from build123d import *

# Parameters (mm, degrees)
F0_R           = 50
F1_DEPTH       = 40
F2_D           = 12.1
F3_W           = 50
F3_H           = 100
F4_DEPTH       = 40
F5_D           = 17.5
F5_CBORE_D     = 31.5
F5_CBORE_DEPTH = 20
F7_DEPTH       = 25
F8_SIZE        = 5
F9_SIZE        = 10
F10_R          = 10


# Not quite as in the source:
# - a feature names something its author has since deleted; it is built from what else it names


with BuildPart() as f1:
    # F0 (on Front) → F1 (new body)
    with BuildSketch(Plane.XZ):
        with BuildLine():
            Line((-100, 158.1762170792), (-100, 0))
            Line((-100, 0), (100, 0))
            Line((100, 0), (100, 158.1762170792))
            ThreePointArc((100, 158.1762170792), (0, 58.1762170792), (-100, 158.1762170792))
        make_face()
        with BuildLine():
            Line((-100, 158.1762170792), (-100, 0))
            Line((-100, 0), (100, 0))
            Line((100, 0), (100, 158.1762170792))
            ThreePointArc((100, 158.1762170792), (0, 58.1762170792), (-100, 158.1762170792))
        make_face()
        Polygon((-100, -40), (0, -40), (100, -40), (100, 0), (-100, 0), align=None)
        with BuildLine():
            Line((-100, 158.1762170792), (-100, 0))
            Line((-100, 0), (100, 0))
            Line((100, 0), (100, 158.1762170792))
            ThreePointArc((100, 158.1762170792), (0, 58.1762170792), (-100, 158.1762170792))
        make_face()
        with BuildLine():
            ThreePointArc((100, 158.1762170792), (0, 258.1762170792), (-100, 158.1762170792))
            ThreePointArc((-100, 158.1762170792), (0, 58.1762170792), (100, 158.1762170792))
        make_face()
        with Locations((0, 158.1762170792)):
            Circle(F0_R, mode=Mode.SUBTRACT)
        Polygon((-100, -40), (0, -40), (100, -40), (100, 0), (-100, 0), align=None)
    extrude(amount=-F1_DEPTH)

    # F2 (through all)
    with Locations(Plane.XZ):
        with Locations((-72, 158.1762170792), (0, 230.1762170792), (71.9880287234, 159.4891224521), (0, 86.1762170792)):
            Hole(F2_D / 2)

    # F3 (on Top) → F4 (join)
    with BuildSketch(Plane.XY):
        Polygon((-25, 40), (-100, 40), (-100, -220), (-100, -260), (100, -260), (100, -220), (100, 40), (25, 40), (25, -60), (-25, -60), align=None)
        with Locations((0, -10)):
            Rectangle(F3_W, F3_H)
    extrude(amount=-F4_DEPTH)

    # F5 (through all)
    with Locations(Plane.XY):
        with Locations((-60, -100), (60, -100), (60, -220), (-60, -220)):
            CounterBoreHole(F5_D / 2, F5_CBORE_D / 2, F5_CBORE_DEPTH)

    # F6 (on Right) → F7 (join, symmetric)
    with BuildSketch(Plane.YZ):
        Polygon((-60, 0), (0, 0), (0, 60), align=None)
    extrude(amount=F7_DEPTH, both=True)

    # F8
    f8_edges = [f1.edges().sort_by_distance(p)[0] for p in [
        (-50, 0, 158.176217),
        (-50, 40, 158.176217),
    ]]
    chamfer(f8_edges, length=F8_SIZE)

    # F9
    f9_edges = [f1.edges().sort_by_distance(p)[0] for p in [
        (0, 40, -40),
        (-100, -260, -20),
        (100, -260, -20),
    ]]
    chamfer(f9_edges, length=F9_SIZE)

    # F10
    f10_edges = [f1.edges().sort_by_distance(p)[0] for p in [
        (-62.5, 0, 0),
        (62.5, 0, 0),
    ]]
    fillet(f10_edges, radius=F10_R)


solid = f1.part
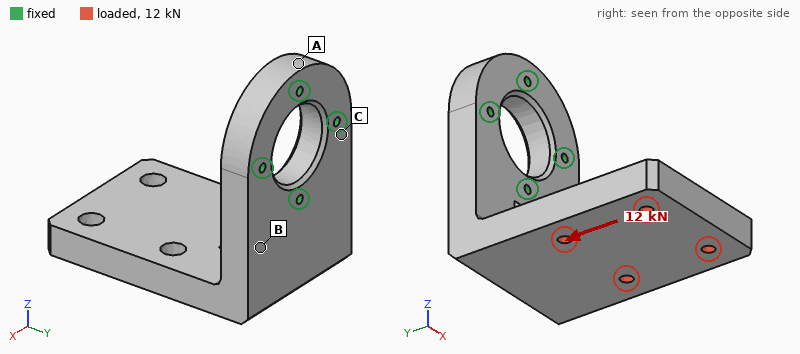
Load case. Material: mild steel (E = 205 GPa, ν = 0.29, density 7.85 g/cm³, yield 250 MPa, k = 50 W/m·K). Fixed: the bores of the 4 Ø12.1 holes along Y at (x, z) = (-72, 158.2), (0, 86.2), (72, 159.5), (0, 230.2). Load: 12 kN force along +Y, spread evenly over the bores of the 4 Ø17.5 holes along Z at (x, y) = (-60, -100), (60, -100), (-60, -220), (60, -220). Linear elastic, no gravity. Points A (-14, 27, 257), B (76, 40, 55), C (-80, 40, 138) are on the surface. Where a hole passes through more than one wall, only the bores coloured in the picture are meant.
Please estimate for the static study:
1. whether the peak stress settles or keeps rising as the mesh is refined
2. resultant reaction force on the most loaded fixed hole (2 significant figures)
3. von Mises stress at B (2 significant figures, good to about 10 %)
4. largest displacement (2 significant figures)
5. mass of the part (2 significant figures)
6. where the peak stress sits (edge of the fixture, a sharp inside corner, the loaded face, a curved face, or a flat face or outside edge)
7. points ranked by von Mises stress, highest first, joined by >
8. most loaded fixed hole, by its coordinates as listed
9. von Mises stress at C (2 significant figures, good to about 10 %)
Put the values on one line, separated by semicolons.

keeps rising; 19 kN; 14 MPa; 0.15 mm; 31 kg; edge of the fixture; B > C > A; (0, 86.2); 11 MPa
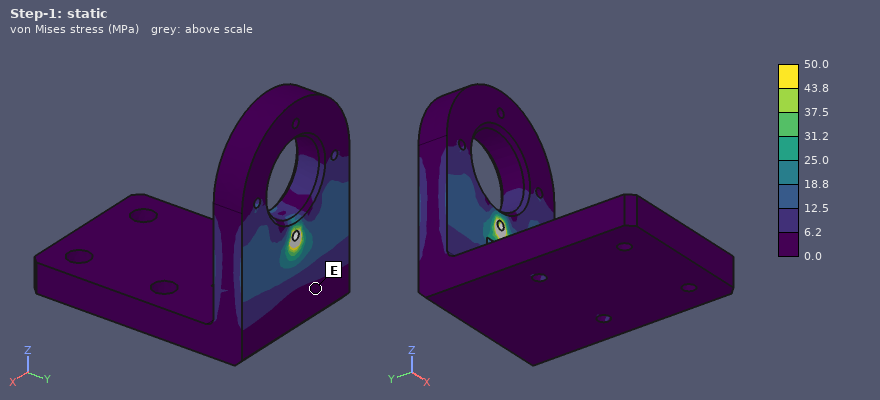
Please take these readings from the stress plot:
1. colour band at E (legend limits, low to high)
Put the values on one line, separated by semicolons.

0.0 to 6.2 MPa
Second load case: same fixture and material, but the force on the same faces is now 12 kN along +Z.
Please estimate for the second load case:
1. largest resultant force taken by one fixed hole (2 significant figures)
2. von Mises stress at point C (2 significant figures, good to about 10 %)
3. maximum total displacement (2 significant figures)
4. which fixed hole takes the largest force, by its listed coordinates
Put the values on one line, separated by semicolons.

17 kN; 13 MPa; 0.38 mm; (0, 86.2)
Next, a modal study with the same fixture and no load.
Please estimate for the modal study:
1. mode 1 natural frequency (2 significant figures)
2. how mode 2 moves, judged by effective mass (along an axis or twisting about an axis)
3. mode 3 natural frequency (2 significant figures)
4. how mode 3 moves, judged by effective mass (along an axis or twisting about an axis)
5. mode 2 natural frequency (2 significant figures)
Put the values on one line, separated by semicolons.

290 Hz; along X; 980 Hz; along Y; 400 Hz
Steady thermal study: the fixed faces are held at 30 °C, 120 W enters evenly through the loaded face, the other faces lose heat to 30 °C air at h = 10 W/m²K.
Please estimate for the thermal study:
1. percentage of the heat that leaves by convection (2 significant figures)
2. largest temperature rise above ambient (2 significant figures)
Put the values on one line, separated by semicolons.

51 %; 53 K
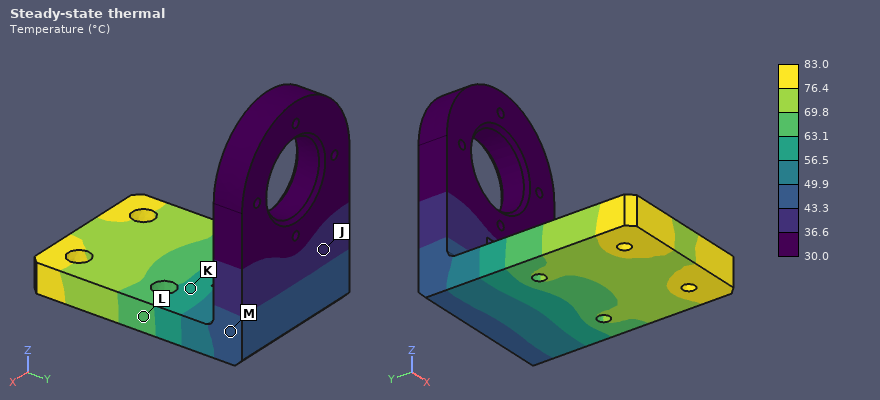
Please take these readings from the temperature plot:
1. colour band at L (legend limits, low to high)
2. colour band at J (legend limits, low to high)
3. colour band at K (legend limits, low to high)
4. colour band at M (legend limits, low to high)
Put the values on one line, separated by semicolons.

63.1 to 69.8 °C; 36.6 to 43.3 °C; 56.5 to 63.1 °C; 43.3 to 49.9 °C
